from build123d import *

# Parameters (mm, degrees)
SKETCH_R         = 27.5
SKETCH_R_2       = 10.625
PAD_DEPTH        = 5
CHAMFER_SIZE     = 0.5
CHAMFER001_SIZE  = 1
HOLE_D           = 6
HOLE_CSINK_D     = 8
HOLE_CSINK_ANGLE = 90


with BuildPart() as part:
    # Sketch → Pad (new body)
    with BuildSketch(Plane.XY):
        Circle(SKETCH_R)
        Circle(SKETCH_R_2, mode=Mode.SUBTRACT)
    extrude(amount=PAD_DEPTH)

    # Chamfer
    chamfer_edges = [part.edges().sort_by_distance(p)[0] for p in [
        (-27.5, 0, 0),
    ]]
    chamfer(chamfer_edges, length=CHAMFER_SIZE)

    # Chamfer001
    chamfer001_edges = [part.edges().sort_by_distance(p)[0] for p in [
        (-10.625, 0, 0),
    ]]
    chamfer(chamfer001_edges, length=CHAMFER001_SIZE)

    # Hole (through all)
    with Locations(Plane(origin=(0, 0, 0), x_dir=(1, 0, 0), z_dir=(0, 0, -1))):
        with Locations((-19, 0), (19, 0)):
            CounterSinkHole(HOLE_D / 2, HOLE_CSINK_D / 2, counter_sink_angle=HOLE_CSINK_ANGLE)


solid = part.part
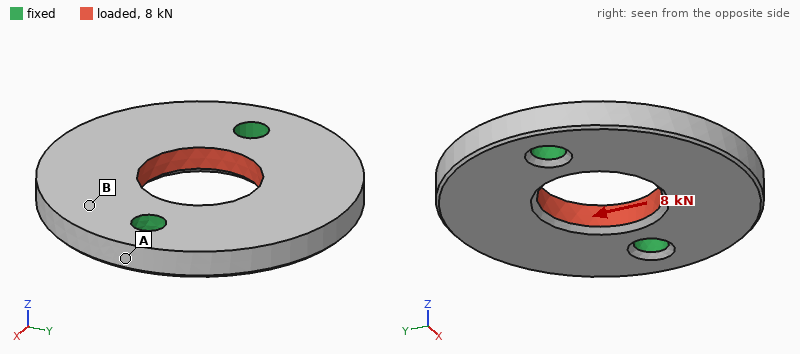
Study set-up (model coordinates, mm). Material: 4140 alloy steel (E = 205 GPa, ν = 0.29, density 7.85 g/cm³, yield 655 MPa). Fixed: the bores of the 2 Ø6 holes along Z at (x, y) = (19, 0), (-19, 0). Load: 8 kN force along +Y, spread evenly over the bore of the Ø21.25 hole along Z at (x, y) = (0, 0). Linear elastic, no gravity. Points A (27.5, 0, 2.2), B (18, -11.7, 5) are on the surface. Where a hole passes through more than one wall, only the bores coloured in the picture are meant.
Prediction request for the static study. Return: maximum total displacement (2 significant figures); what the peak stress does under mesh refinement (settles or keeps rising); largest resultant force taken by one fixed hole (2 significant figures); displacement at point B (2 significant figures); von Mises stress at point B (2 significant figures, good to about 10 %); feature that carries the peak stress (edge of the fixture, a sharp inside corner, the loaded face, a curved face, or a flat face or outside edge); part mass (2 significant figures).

6.5 µm
keeps rising
4.0 kN
1.9 µm
27 MPa
edge of the fixture
77 g
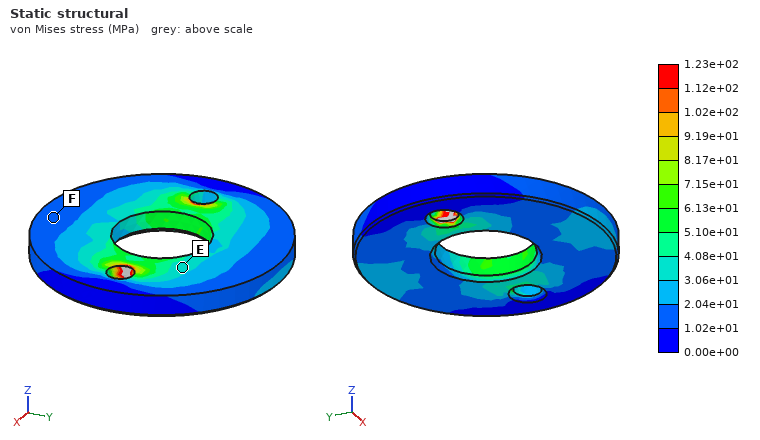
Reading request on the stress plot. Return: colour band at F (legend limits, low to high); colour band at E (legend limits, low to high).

1.02e+01 to 2.04e+01 MPa
3.06e+01 to 4.08e+01 MPa
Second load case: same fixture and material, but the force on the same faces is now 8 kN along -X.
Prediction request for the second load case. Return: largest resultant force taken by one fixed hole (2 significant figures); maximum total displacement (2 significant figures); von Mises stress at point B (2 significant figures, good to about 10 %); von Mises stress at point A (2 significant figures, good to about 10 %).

4.0 kN
4.9 µm
17 MPa
37 MPa
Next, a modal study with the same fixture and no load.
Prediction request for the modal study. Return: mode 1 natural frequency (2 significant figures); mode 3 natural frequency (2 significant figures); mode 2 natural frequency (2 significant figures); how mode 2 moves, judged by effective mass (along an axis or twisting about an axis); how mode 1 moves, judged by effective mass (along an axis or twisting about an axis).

5400 Hz
13 kHz
5700 Hz
along Z
twisting about X
